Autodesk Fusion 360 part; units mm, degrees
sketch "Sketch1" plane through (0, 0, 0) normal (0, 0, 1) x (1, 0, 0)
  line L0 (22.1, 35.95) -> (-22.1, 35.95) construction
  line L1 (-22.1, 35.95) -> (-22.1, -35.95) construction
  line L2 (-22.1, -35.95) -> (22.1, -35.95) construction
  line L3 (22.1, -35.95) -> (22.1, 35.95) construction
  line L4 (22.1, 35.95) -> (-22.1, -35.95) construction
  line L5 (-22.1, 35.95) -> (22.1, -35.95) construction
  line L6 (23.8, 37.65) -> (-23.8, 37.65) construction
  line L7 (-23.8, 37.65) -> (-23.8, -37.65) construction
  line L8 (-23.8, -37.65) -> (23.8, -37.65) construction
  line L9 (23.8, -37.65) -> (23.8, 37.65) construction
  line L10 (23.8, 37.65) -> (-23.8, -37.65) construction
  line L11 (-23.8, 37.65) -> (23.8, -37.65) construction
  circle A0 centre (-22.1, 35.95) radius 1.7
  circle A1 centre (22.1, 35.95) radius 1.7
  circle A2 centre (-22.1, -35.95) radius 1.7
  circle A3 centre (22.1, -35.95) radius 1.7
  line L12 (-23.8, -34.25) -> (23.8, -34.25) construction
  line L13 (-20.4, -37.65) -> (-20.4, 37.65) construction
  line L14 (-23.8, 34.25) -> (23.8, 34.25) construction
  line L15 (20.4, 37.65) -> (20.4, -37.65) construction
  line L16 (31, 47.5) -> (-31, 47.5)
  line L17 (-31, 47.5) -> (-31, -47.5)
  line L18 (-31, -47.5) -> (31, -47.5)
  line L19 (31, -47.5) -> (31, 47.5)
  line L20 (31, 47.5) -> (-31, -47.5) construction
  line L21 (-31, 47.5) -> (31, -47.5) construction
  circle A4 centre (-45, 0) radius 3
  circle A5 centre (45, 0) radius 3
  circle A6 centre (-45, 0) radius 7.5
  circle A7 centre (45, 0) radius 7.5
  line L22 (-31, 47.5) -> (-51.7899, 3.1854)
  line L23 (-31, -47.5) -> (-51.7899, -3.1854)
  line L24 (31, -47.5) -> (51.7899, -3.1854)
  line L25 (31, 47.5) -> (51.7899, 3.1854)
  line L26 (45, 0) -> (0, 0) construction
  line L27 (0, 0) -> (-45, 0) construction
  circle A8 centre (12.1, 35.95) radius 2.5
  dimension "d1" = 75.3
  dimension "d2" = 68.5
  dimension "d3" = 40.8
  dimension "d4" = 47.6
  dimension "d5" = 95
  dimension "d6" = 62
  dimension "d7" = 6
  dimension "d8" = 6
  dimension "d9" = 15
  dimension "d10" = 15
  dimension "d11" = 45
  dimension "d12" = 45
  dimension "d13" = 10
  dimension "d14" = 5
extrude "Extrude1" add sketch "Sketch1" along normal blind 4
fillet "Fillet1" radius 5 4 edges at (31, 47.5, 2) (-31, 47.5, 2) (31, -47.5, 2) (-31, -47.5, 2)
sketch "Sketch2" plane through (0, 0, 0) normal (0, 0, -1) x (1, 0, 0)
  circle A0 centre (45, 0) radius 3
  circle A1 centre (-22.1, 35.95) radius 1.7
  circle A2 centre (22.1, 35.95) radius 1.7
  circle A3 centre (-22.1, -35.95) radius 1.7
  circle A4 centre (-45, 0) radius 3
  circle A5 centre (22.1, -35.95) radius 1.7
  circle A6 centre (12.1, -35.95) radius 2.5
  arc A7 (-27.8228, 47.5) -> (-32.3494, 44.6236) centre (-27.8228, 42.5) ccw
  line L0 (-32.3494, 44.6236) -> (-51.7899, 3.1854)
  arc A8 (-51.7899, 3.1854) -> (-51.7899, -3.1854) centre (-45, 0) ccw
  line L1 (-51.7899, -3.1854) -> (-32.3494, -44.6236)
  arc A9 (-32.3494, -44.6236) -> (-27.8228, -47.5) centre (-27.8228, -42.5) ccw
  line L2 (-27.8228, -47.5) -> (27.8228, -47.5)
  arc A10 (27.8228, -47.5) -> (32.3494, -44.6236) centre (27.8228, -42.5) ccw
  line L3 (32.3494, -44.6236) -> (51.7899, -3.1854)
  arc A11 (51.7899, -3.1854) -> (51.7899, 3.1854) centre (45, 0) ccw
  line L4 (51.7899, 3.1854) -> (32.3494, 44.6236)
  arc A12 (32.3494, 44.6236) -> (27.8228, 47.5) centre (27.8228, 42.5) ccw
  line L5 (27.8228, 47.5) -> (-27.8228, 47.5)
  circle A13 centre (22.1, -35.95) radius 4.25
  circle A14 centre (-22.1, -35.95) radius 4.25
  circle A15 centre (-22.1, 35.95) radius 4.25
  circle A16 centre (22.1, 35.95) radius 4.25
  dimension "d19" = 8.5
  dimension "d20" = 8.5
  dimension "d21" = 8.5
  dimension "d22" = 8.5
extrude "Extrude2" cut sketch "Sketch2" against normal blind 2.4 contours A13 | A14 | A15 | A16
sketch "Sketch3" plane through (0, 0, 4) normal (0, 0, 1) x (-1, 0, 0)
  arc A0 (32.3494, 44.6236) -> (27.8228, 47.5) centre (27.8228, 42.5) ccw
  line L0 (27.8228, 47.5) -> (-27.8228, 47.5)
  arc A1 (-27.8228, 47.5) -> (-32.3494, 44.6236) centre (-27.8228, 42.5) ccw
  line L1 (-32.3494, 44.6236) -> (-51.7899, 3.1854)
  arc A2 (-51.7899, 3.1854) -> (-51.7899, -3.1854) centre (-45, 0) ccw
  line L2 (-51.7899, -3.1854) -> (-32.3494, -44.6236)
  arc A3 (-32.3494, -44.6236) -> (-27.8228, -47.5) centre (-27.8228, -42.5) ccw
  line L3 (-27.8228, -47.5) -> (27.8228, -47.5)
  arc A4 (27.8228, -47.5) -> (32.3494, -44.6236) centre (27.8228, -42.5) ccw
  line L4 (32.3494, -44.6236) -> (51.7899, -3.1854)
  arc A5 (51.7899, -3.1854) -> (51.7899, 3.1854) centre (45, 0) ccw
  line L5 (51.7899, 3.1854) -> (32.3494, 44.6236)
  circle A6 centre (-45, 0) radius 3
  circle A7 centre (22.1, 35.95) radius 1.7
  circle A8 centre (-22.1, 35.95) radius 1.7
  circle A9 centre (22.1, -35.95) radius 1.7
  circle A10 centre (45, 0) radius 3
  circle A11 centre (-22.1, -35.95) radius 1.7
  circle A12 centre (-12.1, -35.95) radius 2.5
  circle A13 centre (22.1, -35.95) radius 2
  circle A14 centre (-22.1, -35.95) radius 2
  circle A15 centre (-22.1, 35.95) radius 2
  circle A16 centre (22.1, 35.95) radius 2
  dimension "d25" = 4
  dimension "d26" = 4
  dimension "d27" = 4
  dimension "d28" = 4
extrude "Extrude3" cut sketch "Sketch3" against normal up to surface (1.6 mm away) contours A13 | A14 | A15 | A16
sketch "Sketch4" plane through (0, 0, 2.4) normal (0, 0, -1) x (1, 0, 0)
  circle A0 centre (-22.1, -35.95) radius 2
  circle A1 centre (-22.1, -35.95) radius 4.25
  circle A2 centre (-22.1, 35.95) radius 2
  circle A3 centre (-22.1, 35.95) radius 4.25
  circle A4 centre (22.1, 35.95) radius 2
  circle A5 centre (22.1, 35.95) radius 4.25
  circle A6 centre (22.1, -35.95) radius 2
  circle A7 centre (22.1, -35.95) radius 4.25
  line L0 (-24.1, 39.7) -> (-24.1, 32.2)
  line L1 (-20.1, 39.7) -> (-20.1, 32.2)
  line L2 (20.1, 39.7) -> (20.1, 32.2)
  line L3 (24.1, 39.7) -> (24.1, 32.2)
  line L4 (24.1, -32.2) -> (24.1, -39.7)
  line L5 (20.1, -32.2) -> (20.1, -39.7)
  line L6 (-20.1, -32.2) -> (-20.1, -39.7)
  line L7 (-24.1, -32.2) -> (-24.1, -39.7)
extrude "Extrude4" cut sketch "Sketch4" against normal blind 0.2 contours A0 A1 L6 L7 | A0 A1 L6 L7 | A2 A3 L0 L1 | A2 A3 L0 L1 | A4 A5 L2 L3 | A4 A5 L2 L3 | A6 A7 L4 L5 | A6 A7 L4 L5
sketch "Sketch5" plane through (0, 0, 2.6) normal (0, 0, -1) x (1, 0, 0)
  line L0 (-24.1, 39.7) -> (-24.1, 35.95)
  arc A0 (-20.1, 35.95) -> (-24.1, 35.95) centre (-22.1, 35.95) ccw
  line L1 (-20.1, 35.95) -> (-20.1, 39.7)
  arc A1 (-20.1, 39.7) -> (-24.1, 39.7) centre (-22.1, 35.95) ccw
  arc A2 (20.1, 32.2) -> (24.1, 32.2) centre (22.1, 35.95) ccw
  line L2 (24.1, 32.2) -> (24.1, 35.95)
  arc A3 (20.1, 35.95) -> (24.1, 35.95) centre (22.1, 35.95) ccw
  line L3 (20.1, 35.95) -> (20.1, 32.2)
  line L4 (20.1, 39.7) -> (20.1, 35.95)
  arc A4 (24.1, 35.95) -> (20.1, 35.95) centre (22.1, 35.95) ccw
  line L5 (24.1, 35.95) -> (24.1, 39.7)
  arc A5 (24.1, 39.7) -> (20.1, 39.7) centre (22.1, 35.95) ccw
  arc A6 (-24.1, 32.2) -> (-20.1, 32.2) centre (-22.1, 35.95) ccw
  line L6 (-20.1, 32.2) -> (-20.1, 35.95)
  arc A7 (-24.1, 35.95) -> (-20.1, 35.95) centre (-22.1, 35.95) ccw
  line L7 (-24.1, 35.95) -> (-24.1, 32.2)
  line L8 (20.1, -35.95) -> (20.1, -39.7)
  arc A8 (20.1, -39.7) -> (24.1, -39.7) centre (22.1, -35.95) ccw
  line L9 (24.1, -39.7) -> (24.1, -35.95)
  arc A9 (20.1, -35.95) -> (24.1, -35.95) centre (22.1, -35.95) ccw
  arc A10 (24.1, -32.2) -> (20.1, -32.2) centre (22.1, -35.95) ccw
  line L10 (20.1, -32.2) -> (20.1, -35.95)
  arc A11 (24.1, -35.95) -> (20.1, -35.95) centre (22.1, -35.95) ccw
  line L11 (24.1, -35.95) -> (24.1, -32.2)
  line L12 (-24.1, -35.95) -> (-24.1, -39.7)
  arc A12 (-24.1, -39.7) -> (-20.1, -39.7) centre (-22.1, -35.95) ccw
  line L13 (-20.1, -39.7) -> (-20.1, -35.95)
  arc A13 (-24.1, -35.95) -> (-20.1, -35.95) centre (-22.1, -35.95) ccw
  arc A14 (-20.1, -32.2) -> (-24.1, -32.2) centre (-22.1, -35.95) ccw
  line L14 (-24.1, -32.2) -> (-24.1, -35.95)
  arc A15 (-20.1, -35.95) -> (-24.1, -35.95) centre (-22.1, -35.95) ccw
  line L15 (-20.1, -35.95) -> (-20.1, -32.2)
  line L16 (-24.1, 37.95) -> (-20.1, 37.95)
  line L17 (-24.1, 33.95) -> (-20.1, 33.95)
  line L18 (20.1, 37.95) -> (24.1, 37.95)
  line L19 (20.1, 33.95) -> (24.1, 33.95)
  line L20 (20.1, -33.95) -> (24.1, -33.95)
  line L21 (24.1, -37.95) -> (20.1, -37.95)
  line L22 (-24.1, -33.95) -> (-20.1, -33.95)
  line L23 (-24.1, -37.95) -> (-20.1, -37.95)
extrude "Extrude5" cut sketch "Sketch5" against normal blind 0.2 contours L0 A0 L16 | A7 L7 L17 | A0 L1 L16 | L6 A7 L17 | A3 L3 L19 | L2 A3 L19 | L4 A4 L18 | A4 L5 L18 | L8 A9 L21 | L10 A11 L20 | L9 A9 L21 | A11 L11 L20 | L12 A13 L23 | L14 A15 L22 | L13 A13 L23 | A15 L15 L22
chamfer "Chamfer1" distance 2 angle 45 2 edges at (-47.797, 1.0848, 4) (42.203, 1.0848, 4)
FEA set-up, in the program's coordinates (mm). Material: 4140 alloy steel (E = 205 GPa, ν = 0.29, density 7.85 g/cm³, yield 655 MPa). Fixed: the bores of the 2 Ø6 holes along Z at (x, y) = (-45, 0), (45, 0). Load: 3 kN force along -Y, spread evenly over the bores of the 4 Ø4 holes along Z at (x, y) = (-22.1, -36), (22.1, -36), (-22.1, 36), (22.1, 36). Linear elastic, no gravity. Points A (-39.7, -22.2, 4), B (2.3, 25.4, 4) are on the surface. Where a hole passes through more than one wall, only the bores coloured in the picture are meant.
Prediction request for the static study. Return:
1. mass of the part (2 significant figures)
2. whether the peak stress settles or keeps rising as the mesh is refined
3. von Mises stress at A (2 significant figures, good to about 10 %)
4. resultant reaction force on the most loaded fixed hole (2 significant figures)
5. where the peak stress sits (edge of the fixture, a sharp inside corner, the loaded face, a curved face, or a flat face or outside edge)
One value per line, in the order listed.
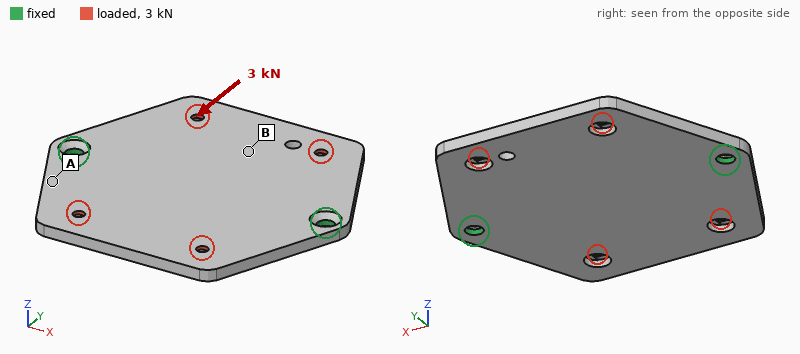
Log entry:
240 g
keeps rising
22 MPa
1.5 kN
edge of the fixture
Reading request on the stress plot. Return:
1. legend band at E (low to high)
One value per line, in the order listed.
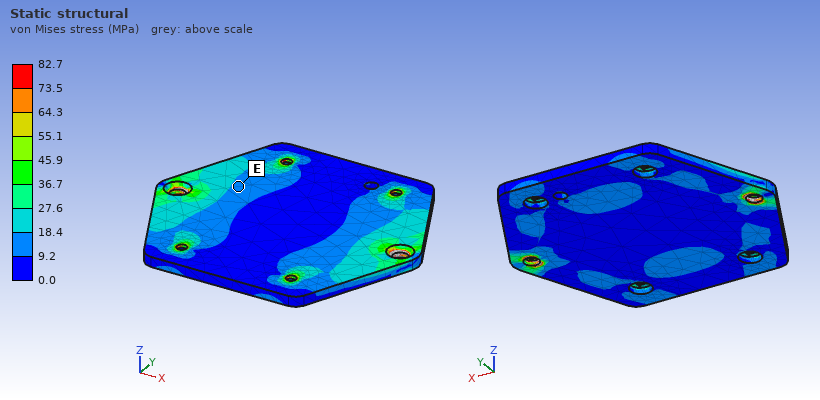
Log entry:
9.2 to 18.4 MPa
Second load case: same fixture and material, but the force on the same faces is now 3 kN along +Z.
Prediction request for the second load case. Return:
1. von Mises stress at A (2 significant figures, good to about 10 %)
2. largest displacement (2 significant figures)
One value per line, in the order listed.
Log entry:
110 MPa
0.49 mm
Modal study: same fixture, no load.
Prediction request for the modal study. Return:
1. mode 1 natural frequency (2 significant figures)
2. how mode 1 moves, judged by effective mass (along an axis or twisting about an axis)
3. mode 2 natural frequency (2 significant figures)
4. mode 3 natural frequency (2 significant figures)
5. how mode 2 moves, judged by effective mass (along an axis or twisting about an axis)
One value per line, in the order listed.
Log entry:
850 Hz
twisting about X
1300 Hz
2700 Hz
along Z
